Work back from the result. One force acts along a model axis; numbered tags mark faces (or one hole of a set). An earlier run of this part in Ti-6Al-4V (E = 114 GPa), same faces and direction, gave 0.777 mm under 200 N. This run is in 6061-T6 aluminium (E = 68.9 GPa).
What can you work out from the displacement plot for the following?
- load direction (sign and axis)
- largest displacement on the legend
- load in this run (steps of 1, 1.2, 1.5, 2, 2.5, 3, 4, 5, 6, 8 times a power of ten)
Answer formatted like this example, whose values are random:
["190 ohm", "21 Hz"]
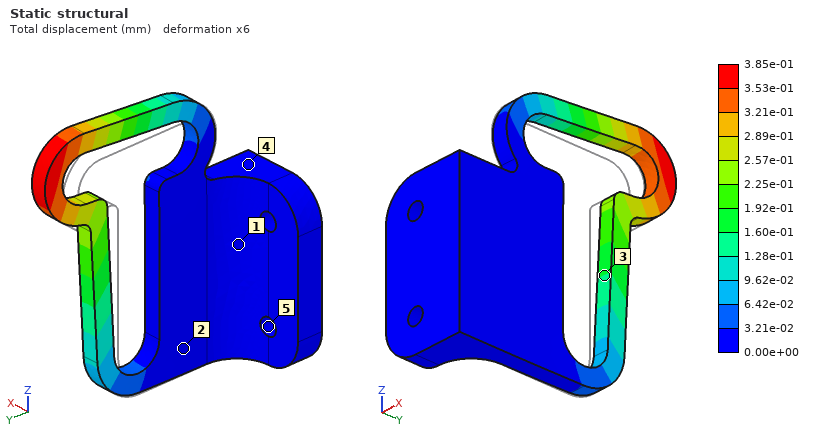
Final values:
["+X", "3.85e-01 mm", "60 N"]
